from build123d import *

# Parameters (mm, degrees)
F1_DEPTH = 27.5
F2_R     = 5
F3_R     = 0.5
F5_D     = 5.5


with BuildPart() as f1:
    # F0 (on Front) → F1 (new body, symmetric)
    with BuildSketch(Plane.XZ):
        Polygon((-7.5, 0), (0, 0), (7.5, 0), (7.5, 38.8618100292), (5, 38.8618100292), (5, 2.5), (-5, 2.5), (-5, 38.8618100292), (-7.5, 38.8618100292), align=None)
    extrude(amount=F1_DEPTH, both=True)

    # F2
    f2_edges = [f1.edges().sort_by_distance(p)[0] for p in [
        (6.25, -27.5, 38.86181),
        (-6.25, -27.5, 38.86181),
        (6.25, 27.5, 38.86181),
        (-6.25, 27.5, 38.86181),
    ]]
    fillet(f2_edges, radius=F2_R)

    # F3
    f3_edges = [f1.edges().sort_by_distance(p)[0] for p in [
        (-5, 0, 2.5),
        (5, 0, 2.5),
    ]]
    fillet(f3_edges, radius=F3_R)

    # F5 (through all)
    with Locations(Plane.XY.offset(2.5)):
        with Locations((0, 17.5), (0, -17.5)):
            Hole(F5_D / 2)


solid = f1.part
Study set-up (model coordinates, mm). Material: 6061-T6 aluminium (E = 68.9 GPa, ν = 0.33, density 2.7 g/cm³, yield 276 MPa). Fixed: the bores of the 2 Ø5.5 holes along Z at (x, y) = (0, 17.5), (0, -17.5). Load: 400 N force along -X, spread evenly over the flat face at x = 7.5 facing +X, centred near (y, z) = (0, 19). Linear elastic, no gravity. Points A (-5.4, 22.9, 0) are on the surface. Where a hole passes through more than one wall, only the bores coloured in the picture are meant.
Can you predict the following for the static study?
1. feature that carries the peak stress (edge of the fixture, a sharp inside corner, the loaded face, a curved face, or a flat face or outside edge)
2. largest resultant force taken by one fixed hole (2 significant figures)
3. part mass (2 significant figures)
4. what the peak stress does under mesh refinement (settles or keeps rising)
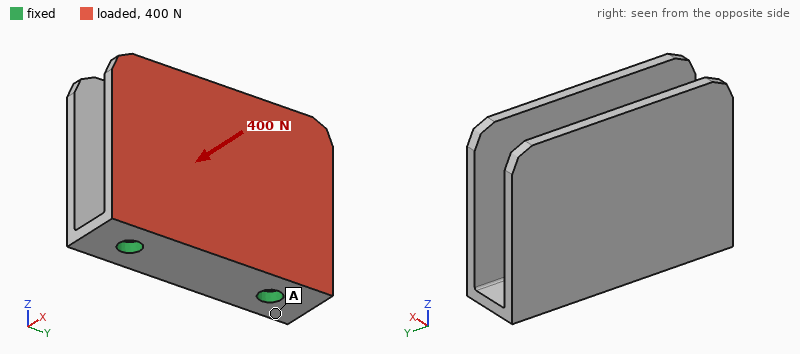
edge of the fixture
200 N
32 g
keeps rising
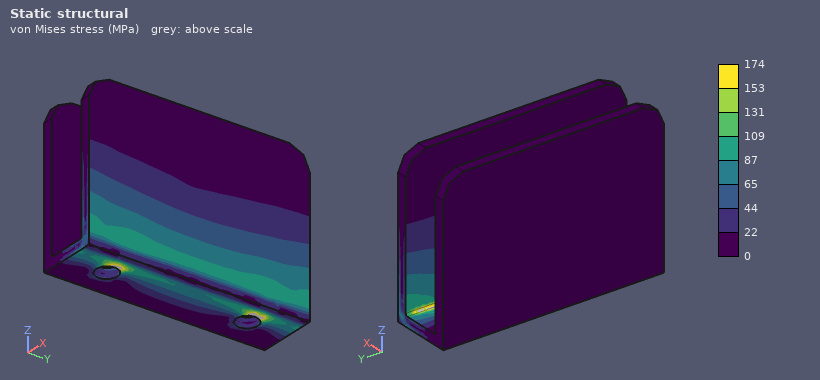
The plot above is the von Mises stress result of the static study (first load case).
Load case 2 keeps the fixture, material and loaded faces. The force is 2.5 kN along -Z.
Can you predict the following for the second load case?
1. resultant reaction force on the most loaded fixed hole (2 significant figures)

1.3 kN
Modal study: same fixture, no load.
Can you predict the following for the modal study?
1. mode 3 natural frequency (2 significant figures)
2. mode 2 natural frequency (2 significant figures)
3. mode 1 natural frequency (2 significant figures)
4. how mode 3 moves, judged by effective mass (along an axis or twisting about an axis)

2500 Hz
1300 Hz
1200 Hz
twisting about Z
